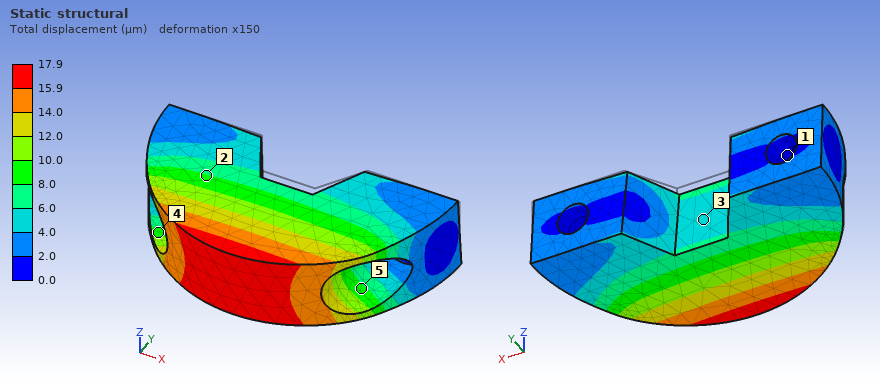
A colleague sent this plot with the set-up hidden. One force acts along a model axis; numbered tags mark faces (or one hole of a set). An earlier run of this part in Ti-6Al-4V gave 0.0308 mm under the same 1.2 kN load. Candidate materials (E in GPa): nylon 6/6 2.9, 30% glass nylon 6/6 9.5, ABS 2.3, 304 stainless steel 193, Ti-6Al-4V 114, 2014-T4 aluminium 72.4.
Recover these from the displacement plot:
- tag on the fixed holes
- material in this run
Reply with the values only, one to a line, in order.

1
304 stainless steel
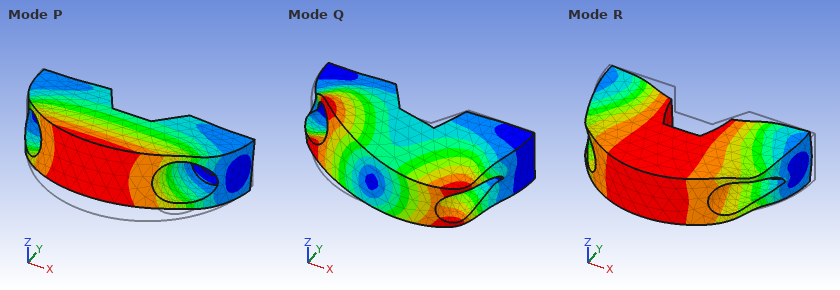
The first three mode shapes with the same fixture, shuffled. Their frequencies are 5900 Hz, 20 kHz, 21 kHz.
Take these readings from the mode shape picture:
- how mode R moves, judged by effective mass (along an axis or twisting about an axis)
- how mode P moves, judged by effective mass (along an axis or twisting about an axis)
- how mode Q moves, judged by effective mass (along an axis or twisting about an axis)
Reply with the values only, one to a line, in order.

along Y
along Z
twisting about Y
